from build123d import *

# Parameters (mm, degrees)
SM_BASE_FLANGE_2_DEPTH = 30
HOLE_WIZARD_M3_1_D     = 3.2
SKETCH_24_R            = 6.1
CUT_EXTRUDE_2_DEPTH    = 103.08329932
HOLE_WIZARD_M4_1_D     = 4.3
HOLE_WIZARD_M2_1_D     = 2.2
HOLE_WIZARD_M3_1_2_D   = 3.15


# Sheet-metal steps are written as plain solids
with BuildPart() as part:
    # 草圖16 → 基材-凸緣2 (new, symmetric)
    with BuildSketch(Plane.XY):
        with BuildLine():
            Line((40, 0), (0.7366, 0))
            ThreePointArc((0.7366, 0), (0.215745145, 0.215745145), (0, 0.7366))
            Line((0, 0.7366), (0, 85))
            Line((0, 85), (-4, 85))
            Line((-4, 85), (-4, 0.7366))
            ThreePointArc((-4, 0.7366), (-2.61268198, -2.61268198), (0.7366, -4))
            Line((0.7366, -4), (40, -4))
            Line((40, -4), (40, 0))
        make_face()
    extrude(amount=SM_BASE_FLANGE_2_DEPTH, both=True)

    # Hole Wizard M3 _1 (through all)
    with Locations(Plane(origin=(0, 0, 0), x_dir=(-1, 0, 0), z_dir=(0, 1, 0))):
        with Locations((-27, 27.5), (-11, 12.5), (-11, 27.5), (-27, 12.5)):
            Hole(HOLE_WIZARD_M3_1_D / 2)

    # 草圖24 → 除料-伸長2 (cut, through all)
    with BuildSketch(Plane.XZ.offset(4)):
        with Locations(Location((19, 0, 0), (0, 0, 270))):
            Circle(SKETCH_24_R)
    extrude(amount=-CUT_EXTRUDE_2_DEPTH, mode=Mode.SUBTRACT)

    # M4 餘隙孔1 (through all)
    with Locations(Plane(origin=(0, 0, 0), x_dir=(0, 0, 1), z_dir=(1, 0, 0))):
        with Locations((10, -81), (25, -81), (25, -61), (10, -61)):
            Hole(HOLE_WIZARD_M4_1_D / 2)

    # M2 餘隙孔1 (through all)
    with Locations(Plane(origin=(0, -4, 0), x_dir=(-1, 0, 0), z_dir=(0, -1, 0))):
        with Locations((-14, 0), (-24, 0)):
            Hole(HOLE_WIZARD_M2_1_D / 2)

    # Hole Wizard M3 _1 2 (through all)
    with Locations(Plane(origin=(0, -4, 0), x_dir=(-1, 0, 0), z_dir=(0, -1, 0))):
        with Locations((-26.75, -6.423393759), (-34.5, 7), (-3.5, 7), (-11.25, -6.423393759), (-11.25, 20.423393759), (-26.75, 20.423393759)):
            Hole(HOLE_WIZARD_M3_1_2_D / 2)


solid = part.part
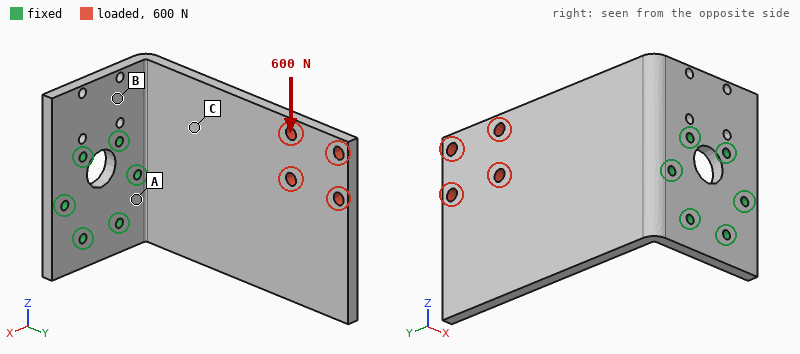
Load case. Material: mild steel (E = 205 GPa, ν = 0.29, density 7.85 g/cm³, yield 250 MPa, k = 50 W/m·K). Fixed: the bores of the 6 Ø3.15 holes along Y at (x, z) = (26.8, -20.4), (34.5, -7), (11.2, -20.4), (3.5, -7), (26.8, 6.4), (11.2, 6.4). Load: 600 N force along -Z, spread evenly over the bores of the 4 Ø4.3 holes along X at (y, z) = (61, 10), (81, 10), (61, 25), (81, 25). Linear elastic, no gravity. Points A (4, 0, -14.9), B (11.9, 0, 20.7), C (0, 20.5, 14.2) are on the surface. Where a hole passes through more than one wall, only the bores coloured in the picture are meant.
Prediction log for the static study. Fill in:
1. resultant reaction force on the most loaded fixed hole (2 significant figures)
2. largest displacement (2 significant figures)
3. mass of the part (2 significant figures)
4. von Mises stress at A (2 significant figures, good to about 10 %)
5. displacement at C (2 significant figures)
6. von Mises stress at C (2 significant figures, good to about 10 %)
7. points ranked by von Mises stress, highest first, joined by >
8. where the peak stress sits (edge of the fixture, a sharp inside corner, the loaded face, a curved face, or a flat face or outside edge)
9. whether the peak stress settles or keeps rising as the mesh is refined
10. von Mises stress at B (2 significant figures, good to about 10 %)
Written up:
1.3 kN
0.20 mm
230 g
93 MPa
0.062 mm
23 MPa
A > B > C
edge of the fixture
keeps rising
58 MPa
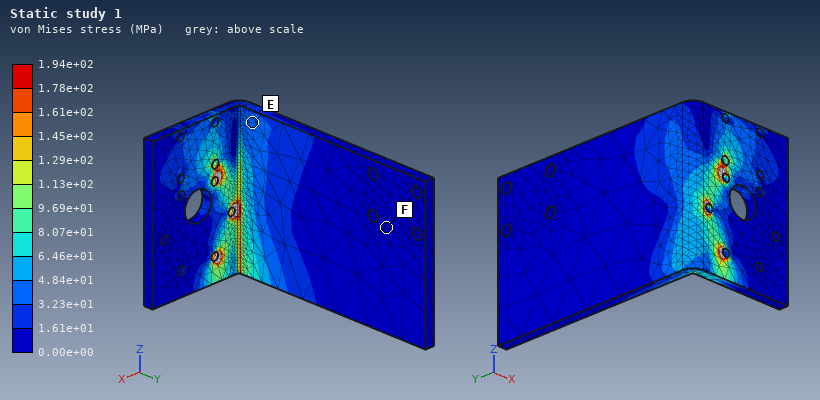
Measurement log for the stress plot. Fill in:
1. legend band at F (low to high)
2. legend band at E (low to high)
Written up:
0.00e+00 to 1.61e+01 MPa
3.23e+01 to 4.84e+01 MPa
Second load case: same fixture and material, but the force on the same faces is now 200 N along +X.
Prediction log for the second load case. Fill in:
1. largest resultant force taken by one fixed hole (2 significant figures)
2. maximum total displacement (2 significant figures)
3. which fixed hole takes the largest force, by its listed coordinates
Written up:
820 N
0.72 mm
(3.5, -7)
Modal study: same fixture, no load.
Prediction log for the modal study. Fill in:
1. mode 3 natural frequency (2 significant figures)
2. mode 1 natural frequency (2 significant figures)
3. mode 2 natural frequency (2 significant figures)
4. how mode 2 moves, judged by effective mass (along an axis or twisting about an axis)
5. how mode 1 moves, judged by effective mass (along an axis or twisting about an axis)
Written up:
1500 Hz
390 Hz
1100 Hz
along Z
along X
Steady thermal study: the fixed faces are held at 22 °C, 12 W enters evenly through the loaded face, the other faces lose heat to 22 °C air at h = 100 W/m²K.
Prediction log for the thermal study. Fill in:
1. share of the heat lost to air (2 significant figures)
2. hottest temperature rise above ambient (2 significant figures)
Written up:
91 %
36 K
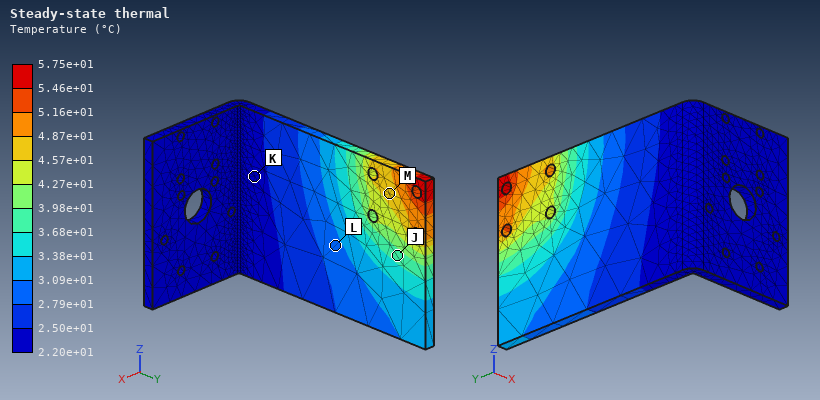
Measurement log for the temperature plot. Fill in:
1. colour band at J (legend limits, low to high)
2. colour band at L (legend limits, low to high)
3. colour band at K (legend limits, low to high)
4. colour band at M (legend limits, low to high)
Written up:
3.68e+01 to 3.98e+01 °C
2.79e+01 to 3.09e+01 °C
2.20e+01 to 2.50e+01 °C
4.57e+01 to 4.87e+01 °C
